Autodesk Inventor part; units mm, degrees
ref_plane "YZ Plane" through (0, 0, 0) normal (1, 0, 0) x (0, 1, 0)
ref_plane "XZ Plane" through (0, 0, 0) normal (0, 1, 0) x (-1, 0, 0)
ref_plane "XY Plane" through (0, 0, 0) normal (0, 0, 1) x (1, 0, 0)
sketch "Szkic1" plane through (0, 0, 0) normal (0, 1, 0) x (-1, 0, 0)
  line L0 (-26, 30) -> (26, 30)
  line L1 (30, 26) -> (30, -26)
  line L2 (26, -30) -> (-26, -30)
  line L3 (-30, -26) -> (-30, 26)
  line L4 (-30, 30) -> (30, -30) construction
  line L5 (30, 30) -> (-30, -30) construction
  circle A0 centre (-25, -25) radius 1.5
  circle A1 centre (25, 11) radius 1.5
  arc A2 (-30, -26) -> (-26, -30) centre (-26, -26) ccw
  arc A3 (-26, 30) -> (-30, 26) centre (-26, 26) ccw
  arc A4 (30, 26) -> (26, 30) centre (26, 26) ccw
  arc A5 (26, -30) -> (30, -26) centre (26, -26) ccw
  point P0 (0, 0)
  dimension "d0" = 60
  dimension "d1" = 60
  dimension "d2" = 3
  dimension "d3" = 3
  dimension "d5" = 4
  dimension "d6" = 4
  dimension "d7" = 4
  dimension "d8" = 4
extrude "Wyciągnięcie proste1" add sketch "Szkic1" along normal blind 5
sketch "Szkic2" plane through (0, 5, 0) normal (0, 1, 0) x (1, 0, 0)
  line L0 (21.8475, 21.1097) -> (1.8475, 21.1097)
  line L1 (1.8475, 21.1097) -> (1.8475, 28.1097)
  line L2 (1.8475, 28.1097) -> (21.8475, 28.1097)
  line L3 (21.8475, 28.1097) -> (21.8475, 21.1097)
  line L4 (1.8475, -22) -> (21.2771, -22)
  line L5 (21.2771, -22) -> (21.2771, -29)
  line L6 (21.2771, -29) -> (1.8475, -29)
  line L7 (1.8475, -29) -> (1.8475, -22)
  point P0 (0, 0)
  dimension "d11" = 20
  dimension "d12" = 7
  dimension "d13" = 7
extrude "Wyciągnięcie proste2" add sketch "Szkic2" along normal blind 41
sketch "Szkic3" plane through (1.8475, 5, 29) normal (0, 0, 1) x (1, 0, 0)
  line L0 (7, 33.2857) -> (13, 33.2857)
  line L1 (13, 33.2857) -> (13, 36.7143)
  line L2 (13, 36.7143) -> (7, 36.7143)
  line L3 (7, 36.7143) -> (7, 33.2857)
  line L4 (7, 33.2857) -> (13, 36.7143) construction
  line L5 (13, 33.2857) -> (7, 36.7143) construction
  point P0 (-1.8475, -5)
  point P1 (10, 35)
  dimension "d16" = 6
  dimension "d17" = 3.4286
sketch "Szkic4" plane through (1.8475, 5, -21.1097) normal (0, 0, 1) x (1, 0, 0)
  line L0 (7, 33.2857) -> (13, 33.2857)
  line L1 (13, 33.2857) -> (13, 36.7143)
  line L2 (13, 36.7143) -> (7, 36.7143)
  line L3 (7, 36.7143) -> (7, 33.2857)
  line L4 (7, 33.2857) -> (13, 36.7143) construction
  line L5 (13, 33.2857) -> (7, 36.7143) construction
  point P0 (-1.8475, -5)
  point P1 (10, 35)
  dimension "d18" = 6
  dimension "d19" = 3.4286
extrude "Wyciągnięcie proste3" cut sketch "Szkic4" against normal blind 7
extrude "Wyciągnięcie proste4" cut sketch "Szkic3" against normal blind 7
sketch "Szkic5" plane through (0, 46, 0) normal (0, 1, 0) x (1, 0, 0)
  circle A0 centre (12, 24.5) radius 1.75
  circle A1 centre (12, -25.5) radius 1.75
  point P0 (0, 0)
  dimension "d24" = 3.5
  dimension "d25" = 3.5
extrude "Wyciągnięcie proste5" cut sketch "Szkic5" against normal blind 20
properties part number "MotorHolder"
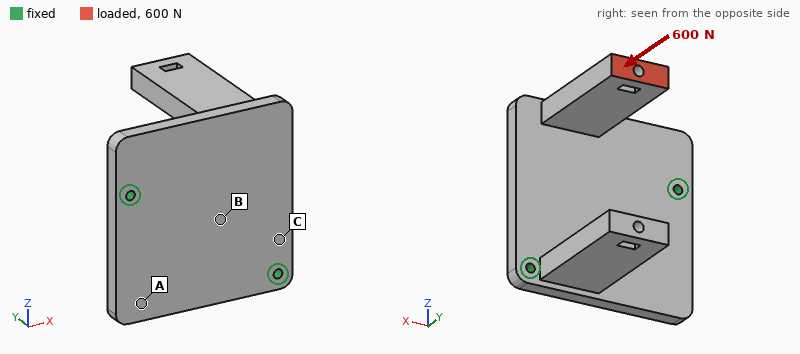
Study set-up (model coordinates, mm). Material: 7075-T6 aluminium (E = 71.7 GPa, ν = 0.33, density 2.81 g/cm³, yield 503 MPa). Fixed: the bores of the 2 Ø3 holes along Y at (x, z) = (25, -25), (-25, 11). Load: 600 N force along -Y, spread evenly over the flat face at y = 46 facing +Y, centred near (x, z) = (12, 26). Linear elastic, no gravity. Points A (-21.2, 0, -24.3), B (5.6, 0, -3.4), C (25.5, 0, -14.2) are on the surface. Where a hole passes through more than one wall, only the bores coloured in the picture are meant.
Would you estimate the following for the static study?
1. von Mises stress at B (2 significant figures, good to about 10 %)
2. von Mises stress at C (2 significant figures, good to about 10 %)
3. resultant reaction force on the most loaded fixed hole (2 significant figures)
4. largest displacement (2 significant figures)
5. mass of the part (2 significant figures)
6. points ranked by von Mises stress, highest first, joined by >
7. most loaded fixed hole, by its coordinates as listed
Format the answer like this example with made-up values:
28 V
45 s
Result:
38 MPa
68 MPa
420 N
0.65 mm
80 g
C > B > A
(-25, 11)
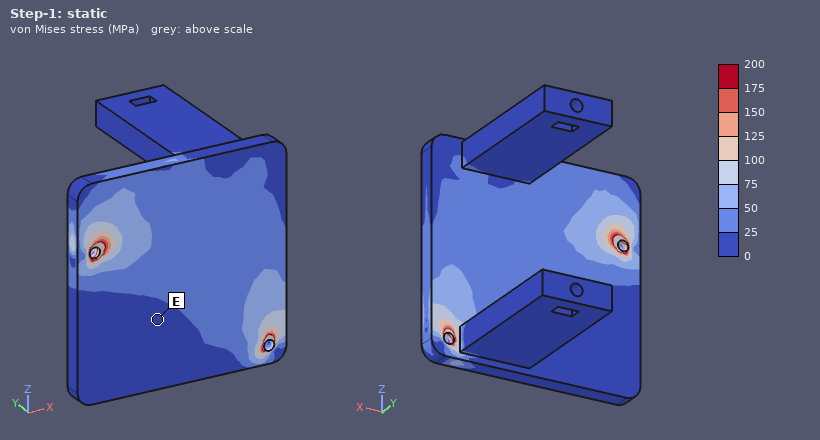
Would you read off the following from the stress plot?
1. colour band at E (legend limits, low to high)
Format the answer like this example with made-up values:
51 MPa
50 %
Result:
0 to 25 MPa
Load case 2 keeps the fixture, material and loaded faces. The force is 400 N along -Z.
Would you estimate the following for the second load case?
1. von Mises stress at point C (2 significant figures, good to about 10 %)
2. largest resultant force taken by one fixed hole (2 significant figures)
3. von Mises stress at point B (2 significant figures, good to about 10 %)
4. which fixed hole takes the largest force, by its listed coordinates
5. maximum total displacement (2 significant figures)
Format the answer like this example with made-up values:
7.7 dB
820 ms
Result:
34 MPa
330 N
31 MPa
(25, -25)
0.97 mm
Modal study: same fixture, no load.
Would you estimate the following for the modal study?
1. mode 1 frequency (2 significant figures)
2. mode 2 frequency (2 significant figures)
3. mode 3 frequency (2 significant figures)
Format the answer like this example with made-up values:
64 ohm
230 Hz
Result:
1100 Hz
2000 Hz
2200 Hz
